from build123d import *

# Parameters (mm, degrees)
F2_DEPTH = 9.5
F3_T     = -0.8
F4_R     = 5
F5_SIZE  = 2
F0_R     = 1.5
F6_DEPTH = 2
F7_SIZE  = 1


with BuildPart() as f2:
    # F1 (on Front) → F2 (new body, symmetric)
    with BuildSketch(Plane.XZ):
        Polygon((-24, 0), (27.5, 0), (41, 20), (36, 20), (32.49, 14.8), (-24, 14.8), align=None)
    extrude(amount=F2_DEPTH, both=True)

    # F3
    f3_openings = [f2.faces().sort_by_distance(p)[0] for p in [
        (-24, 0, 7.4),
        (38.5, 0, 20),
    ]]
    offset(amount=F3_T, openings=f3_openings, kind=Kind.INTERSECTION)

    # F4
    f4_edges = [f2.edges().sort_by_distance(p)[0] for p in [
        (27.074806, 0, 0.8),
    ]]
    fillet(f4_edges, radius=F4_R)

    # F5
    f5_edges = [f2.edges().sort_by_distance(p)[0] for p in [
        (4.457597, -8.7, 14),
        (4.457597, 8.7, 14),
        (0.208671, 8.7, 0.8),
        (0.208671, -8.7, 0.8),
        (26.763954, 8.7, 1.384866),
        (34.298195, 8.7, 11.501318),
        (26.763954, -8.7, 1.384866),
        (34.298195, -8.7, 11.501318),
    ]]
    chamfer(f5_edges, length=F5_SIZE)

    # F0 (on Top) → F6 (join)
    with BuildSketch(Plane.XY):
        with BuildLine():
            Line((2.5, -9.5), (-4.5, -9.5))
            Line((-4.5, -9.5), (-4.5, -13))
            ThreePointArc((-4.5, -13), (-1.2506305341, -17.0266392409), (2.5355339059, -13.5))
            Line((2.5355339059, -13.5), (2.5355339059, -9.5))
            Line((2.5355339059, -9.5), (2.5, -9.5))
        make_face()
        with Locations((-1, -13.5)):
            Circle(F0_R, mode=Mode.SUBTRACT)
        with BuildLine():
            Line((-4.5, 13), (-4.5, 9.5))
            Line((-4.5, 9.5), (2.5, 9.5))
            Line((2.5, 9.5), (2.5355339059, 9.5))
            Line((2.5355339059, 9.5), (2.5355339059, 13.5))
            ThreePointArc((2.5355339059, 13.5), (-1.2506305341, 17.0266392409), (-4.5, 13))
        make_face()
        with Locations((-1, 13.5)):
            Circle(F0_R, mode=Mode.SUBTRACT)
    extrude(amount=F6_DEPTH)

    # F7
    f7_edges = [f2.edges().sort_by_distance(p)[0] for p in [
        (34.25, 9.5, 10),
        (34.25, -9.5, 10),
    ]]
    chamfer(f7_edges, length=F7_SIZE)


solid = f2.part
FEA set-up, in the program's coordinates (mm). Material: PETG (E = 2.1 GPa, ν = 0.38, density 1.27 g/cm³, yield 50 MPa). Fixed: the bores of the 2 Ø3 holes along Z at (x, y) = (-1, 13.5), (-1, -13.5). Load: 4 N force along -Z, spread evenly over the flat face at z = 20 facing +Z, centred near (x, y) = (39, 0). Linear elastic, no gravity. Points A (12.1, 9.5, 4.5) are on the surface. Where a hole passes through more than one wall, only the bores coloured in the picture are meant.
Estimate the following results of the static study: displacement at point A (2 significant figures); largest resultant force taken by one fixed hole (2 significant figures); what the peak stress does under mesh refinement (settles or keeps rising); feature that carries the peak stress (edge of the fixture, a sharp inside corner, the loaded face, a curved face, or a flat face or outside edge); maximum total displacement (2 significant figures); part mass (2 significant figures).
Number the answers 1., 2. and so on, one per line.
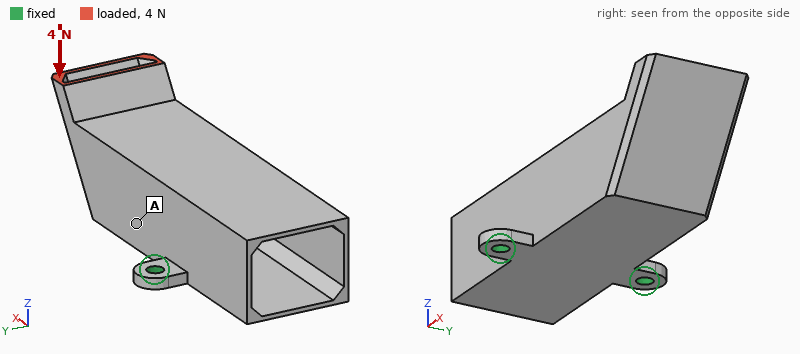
1. 0.25 mm
2. 2.0 N
3. keeps rising
4. edge of the fixture
5. 0.90 mm
6. 5.1 g
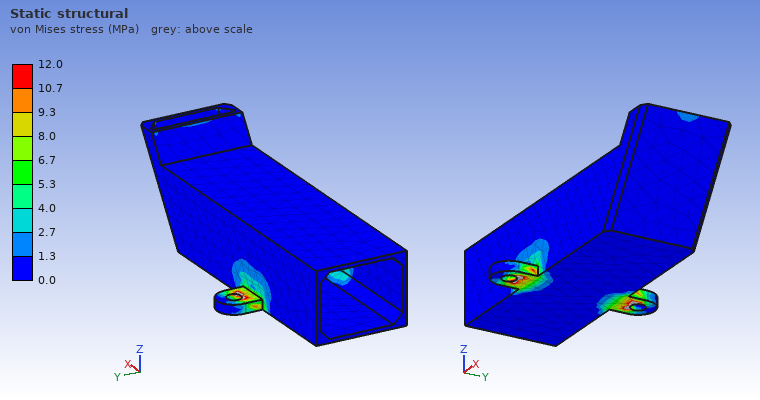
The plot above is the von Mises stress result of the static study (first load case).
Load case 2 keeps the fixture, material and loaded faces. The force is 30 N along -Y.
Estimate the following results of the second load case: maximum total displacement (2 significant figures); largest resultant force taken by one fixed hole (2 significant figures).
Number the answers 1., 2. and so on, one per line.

1. 0.80 mm
2. 61 N
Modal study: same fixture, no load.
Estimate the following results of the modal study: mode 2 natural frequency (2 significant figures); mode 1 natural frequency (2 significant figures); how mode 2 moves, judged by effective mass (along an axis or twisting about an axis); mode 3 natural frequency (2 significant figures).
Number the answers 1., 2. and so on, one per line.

1. 790 Hz
2. 300 Hz
3. along Y
4. 1400 Hz
